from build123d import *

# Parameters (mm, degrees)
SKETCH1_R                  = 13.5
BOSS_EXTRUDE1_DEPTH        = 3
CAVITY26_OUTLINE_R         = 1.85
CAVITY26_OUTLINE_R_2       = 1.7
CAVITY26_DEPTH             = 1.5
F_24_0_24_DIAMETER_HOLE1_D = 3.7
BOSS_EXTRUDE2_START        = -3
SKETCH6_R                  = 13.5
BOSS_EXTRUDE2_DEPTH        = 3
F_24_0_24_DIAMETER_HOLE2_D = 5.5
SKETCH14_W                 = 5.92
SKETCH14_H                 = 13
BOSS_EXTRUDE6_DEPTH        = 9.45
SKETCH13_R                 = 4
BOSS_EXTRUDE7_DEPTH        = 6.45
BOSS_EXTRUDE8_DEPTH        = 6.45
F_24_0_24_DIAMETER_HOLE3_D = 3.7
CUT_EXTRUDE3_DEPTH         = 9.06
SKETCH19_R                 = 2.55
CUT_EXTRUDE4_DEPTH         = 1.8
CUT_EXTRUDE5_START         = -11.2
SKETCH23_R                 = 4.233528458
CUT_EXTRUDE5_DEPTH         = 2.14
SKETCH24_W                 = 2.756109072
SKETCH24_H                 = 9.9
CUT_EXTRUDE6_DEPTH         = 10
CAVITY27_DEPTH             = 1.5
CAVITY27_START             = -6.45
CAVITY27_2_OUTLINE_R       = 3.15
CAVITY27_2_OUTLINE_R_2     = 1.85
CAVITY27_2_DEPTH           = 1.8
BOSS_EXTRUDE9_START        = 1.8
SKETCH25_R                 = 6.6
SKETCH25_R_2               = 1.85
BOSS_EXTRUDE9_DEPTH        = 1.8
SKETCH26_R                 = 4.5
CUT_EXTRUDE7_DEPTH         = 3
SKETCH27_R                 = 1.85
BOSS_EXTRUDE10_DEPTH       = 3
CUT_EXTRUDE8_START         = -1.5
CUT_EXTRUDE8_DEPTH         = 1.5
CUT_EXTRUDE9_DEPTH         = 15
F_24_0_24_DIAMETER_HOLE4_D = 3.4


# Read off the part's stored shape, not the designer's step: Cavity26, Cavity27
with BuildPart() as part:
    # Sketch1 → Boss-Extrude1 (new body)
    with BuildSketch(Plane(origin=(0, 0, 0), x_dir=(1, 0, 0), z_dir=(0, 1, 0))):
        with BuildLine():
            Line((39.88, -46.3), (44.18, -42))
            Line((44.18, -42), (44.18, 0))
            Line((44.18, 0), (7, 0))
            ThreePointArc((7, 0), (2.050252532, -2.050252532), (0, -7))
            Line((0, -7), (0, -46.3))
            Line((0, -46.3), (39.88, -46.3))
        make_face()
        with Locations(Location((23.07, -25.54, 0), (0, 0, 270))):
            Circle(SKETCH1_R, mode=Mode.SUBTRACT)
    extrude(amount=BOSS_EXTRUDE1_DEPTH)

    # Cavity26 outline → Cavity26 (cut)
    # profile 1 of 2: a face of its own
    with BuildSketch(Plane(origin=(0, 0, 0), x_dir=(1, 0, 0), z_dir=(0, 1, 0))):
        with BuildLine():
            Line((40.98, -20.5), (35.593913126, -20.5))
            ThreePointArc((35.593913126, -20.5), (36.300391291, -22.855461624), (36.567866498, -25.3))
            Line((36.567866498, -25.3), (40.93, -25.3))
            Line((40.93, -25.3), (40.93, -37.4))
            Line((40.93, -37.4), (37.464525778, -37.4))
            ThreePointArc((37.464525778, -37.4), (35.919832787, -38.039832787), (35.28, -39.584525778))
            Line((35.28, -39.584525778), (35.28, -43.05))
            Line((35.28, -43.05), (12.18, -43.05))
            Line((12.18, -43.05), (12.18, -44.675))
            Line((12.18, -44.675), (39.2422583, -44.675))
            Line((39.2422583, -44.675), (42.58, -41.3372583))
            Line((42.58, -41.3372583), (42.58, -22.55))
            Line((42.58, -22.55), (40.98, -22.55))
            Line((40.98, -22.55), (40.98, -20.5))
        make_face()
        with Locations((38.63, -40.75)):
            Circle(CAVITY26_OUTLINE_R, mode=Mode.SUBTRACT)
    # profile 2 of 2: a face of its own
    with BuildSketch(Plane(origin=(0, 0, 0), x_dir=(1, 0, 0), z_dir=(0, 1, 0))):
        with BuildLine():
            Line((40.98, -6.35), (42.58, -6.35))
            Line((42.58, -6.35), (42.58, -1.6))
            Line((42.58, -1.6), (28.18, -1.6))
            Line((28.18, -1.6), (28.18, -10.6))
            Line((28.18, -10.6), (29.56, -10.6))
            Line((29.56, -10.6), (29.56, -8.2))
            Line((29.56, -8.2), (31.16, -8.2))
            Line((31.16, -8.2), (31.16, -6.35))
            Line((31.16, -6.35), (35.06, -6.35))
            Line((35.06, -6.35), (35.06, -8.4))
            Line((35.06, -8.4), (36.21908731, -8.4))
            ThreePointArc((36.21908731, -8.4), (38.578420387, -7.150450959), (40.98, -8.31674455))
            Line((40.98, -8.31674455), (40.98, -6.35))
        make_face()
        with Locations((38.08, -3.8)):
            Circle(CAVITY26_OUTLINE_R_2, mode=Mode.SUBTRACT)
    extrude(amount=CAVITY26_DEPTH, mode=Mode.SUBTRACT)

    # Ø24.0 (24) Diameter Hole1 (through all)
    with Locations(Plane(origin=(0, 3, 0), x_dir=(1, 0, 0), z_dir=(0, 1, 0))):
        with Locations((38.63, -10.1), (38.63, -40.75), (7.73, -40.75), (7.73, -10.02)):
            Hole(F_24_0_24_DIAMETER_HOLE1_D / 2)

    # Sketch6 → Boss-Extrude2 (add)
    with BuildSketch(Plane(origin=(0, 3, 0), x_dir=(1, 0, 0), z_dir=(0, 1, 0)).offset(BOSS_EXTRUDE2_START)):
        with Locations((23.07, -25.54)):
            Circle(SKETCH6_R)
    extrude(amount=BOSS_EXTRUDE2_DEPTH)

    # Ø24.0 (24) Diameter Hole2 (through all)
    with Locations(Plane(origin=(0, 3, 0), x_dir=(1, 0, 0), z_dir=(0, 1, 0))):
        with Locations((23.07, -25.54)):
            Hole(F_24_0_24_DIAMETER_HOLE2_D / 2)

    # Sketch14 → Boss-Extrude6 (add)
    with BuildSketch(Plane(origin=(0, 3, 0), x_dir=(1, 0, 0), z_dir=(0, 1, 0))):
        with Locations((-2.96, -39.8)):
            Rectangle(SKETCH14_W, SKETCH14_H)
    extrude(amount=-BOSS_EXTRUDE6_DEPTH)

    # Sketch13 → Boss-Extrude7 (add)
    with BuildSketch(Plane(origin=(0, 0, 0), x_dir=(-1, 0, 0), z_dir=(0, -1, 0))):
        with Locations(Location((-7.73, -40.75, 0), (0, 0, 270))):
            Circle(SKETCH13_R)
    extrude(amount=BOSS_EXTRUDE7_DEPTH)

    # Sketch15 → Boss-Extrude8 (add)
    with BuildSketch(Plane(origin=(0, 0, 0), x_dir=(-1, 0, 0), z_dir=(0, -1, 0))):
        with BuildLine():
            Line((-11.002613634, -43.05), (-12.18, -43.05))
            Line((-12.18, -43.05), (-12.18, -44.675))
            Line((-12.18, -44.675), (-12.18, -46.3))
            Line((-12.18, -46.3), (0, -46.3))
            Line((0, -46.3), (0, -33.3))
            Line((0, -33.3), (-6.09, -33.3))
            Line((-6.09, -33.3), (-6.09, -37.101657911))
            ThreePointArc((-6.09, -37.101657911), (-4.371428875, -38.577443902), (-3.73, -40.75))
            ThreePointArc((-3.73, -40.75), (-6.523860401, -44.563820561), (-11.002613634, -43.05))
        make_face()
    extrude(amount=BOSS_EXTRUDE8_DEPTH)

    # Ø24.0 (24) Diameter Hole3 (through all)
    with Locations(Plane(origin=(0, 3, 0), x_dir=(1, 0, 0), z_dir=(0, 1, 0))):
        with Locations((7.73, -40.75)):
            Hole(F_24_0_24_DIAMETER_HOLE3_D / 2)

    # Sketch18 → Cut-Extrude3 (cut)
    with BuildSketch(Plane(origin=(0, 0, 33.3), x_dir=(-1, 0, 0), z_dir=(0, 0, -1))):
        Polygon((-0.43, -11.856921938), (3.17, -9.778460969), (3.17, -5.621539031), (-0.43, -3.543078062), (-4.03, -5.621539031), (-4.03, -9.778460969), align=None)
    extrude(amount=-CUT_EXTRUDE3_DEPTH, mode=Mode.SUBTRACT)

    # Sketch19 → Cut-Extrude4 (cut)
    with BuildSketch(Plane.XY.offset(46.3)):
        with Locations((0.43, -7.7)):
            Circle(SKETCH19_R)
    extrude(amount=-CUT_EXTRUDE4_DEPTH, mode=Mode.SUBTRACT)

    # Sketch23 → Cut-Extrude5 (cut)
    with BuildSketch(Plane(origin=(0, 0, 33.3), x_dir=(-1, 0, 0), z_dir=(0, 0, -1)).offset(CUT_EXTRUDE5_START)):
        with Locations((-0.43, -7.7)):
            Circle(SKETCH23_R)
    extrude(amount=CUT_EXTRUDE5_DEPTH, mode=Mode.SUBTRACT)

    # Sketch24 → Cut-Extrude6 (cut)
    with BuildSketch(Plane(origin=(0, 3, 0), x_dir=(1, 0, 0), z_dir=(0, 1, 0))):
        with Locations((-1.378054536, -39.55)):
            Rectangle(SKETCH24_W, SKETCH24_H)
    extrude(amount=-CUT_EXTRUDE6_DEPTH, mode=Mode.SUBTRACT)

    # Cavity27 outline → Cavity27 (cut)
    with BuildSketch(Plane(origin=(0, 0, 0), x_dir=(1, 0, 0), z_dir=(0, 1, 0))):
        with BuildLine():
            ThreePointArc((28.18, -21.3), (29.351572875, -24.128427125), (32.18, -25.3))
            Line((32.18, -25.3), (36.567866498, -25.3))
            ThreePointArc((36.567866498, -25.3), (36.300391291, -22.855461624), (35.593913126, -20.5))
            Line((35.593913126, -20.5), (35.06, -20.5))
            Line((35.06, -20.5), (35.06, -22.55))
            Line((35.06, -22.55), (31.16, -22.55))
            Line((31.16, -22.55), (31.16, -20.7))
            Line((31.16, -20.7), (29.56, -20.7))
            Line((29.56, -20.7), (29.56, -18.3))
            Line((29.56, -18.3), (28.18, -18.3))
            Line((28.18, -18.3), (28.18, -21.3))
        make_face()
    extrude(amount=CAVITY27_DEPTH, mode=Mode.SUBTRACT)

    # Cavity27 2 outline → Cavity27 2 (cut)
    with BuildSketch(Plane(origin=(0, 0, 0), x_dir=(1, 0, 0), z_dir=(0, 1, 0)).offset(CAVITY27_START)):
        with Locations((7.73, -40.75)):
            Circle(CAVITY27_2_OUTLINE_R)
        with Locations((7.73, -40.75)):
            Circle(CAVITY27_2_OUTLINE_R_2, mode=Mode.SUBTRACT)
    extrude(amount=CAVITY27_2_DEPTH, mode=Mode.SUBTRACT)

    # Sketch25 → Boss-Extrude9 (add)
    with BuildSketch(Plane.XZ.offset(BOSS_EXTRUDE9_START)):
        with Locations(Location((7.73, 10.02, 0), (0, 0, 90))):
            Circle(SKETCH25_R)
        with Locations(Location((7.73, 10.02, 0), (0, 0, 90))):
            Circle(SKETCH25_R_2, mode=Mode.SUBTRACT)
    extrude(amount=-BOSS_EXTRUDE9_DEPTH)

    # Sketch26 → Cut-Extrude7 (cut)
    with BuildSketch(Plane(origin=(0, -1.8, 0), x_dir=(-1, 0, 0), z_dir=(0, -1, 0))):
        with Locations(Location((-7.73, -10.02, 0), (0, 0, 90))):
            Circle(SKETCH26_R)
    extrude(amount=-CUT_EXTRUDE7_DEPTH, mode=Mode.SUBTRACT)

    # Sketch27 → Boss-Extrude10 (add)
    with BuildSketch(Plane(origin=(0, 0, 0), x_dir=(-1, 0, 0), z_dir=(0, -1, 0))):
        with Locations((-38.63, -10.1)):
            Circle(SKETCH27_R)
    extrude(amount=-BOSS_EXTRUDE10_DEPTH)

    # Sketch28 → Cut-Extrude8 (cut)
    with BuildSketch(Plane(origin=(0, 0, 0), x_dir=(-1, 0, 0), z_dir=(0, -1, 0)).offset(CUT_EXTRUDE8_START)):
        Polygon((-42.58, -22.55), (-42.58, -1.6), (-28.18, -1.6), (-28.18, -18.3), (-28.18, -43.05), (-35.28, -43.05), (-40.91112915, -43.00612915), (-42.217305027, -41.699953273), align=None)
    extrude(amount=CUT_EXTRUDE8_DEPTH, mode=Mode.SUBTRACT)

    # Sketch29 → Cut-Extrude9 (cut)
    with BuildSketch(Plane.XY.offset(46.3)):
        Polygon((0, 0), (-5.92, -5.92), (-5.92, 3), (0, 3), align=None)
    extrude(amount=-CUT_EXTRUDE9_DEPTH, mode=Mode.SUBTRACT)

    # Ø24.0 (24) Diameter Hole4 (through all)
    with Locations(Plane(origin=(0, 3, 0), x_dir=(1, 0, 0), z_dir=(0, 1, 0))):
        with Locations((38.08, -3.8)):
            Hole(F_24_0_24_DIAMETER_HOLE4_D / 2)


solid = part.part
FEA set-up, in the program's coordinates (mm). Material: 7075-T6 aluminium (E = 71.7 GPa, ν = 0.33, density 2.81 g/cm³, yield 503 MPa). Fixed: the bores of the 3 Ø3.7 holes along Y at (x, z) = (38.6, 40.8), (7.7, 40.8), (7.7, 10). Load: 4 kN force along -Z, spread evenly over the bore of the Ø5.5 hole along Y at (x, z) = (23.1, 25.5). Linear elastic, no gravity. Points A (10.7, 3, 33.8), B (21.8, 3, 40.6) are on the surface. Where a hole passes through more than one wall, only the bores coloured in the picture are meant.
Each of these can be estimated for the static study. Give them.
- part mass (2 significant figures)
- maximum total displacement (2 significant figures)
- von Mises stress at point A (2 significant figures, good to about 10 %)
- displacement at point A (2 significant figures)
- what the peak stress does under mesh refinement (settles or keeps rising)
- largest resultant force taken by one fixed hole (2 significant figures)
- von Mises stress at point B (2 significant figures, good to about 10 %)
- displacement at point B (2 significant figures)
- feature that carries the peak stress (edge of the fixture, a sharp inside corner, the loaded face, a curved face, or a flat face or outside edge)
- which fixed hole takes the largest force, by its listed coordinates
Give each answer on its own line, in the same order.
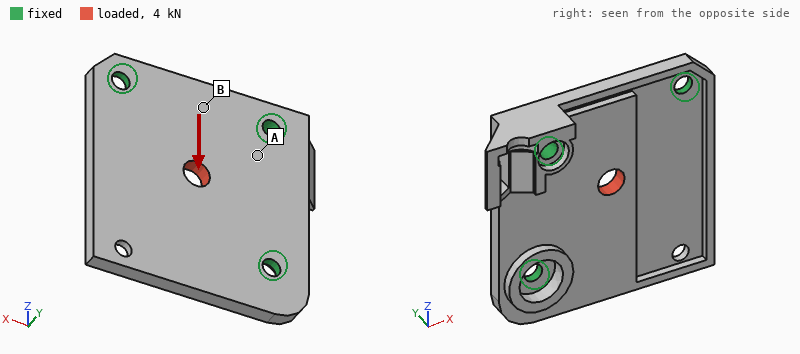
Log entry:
16 g
31 µm
44 MPa
5.2 µm
keeps rising
1.8 kN
19 MPa
14 µm
edge of the fixture
(7.7, 40.8)
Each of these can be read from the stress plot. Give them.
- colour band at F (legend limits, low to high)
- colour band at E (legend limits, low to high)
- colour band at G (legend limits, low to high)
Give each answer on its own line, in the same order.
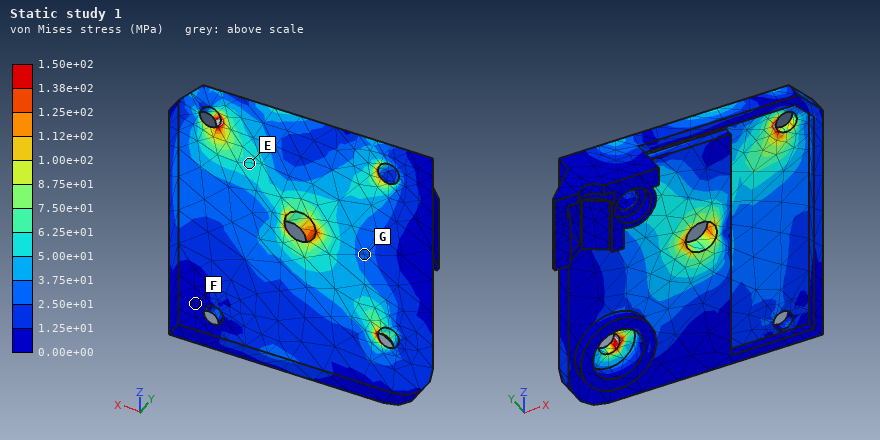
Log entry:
0.00e+00 to 1.25e+01 MPa
5.00e+01 to 6.25e+01 MPa
2.50e+01 to 3.75e+01 MPa
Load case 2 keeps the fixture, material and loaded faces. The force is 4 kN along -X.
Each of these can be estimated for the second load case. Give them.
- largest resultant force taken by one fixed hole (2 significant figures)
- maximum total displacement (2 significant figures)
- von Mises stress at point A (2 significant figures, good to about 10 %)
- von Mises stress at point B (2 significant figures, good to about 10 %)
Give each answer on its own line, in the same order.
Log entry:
1.8 kN
27 µm
44 MPa
12 MPa
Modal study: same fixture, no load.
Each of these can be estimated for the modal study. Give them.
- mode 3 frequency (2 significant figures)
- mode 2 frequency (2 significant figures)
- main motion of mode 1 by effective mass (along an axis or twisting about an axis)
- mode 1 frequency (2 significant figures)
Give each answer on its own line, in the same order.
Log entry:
8200 Hz
8000 Hz
along Y
2800 Hz
